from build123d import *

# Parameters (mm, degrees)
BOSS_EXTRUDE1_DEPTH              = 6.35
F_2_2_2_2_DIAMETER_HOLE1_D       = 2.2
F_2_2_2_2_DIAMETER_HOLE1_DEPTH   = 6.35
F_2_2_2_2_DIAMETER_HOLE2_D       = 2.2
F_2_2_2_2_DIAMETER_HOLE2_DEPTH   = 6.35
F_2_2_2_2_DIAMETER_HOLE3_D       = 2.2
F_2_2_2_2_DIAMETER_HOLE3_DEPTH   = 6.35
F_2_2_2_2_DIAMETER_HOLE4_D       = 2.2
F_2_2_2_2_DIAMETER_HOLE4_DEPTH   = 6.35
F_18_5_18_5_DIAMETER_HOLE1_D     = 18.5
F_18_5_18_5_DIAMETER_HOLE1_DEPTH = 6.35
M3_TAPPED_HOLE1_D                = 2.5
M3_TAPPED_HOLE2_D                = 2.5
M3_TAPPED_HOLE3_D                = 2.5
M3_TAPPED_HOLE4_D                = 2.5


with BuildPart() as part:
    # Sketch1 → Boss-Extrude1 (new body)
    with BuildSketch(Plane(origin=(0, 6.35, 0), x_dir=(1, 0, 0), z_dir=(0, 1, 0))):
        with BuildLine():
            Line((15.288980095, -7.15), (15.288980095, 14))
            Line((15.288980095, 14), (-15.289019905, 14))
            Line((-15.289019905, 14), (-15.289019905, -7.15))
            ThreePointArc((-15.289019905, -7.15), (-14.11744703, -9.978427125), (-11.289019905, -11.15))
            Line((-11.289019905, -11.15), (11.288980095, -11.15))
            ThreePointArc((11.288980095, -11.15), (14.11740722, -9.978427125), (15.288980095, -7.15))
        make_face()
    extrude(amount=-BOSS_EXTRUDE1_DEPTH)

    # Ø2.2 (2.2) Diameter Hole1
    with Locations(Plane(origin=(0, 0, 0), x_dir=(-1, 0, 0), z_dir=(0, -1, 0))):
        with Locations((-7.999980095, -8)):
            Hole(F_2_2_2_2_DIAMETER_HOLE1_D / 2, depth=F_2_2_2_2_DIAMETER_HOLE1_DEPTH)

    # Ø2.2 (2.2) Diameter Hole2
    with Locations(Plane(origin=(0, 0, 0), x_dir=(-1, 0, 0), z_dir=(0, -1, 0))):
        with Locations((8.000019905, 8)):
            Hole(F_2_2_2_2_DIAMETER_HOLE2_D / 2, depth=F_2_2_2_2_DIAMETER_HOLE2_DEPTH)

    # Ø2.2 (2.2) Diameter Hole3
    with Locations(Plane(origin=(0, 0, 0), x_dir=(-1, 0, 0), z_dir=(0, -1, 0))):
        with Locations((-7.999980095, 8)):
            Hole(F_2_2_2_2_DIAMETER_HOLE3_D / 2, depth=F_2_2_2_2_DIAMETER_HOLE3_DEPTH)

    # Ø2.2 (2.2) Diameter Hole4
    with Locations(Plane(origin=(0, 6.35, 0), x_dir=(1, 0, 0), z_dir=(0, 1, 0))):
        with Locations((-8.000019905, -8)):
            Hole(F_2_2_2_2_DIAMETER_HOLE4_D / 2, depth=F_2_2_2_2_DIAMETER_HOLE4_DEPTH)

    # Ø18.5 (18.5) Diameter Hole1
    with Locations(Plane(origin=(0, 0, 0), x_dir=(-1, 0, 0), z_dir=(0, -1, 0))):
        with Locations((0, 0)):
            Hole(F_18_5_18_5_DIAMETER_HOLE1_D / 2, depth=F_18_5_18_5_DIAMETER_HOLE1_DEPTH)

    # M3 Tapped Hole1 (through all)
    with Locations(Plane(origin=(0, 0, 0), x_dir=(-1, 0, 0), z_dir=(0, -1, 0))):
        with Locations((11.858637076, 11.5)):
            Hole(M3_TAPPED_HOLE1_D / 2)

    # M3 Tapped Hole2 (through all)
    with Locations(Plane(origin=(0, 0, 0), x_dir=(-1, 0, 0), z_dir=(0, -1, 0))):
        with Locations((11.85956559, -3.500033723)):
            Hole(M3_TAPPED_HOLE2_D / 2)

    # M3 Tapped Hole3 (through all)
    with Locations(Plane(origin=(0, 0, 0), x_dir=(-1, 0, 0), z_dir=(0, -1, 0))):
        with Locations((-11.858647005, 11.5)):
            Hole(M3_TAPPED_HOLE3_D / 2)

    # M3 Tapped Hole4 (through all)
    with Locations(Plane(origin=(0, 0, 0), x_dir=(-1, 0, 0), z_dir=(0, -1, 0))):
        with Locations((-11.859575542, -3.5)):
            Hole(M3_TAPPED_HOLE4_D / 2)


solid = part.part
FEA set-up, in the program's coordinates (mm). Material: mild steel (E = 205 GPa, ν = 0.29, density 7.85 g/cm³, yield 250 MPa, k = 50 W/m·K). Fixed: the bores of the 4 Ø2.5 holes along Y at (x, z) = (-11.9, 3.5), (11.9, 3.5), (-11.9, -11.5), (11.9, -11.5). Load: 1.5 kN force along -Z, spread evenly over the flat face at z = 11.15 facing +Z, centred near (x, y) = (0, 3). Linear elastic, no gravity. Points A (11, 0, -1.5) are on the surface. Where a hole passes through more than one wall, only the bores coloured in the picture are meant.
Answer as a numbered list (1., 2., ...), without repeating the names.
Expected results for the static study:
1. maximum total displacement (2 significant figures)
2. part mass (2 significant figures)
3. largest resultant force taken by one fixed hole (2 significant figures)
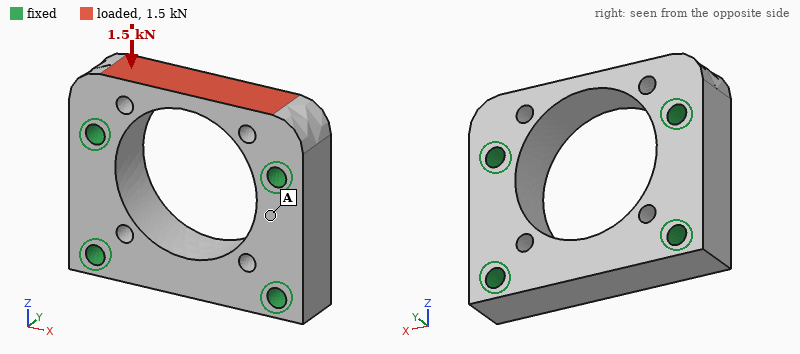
1. 6.4 µm
2. 23 g
3. 870 N
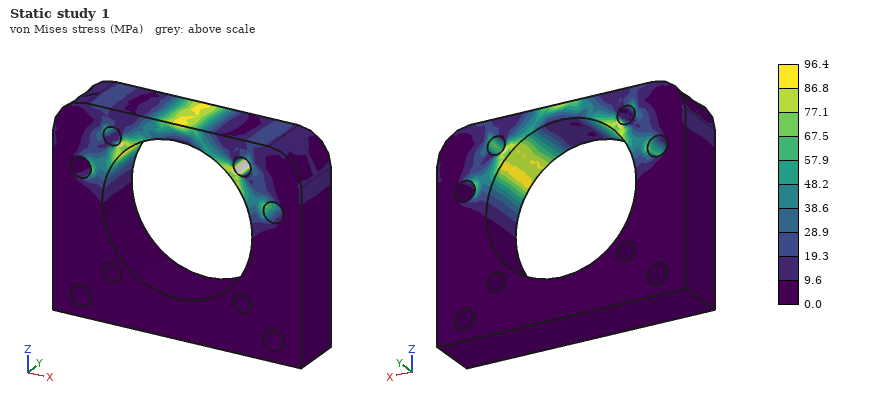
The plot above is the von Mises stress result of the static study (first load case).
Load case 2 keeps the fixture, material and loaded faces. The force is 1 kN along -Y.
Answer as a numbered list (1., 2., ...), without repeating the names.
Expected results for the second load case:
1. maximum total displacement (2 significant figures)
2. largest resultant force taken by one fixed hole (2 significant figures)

1. 10 µm
2. 520 N
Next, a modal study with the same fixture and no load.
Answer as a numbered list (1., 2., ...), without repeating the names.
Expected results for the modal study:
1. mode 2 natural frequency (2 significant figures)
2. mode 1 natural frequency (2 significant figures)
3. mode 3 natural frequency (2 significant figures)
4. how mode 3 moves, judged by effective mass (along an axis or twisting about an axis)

1. 45 kHz
2. 38 kHz
3. 48 kHz
4. along Y
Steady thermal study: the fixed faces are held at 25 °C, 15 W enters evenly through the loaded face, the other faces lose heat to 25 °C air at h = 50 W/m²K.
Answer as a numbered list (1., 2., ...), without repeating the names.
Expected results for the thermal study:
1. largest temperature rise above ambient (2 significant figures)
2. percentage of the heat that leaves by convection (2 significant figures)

1. 49 K
2. 4.2 %
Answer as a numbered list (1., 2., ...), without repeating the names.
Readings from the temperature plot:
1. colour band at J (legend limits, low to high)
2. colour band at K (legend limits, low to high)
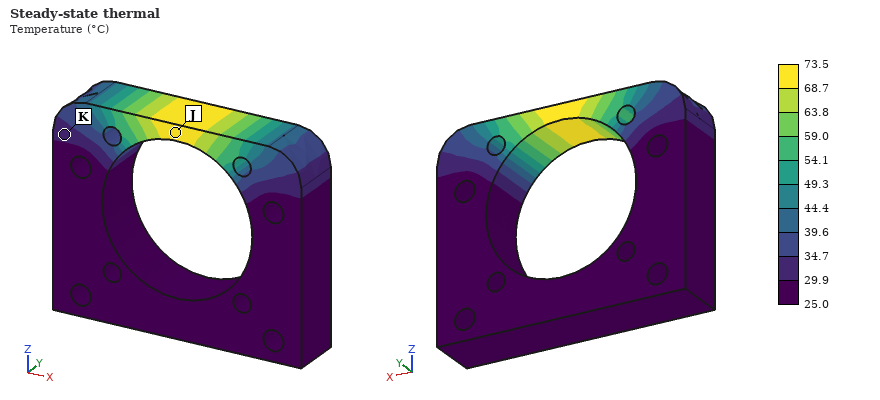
1. 68.7 to 73.5 °C
2. 29.9 to 34.7 °C
